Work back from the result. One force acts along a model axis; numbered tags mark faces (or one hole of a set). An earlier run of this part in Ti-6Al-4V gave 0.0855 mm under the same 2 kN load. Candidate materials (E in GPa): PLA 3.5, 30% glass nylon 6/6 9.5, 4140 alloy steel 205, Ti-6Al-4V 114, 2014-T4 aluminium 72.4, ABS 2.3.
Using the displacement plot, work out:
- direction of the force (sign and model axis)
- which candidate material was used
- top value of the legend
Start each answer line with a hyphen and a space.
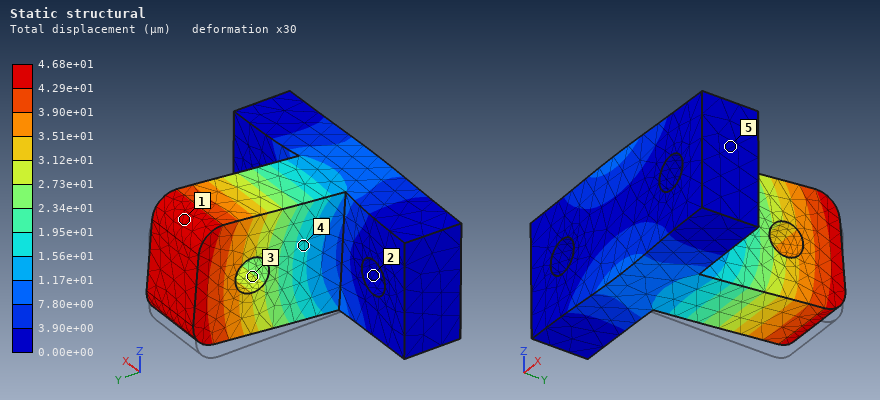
- +Z
- 4140 alloy steel
- 4.68e+01 µm
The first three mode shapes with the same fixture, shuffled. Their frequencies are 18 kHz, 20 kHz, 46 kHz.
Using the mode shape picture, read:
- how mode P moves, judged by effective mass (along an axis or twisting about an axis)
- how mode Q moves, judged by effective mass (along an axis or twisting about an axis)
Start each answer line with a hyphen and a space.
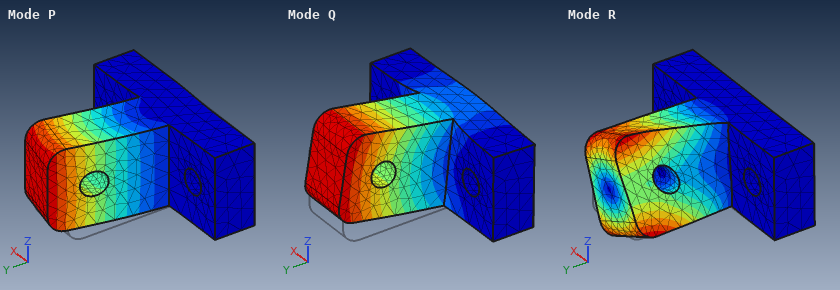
- along X
- along Z
